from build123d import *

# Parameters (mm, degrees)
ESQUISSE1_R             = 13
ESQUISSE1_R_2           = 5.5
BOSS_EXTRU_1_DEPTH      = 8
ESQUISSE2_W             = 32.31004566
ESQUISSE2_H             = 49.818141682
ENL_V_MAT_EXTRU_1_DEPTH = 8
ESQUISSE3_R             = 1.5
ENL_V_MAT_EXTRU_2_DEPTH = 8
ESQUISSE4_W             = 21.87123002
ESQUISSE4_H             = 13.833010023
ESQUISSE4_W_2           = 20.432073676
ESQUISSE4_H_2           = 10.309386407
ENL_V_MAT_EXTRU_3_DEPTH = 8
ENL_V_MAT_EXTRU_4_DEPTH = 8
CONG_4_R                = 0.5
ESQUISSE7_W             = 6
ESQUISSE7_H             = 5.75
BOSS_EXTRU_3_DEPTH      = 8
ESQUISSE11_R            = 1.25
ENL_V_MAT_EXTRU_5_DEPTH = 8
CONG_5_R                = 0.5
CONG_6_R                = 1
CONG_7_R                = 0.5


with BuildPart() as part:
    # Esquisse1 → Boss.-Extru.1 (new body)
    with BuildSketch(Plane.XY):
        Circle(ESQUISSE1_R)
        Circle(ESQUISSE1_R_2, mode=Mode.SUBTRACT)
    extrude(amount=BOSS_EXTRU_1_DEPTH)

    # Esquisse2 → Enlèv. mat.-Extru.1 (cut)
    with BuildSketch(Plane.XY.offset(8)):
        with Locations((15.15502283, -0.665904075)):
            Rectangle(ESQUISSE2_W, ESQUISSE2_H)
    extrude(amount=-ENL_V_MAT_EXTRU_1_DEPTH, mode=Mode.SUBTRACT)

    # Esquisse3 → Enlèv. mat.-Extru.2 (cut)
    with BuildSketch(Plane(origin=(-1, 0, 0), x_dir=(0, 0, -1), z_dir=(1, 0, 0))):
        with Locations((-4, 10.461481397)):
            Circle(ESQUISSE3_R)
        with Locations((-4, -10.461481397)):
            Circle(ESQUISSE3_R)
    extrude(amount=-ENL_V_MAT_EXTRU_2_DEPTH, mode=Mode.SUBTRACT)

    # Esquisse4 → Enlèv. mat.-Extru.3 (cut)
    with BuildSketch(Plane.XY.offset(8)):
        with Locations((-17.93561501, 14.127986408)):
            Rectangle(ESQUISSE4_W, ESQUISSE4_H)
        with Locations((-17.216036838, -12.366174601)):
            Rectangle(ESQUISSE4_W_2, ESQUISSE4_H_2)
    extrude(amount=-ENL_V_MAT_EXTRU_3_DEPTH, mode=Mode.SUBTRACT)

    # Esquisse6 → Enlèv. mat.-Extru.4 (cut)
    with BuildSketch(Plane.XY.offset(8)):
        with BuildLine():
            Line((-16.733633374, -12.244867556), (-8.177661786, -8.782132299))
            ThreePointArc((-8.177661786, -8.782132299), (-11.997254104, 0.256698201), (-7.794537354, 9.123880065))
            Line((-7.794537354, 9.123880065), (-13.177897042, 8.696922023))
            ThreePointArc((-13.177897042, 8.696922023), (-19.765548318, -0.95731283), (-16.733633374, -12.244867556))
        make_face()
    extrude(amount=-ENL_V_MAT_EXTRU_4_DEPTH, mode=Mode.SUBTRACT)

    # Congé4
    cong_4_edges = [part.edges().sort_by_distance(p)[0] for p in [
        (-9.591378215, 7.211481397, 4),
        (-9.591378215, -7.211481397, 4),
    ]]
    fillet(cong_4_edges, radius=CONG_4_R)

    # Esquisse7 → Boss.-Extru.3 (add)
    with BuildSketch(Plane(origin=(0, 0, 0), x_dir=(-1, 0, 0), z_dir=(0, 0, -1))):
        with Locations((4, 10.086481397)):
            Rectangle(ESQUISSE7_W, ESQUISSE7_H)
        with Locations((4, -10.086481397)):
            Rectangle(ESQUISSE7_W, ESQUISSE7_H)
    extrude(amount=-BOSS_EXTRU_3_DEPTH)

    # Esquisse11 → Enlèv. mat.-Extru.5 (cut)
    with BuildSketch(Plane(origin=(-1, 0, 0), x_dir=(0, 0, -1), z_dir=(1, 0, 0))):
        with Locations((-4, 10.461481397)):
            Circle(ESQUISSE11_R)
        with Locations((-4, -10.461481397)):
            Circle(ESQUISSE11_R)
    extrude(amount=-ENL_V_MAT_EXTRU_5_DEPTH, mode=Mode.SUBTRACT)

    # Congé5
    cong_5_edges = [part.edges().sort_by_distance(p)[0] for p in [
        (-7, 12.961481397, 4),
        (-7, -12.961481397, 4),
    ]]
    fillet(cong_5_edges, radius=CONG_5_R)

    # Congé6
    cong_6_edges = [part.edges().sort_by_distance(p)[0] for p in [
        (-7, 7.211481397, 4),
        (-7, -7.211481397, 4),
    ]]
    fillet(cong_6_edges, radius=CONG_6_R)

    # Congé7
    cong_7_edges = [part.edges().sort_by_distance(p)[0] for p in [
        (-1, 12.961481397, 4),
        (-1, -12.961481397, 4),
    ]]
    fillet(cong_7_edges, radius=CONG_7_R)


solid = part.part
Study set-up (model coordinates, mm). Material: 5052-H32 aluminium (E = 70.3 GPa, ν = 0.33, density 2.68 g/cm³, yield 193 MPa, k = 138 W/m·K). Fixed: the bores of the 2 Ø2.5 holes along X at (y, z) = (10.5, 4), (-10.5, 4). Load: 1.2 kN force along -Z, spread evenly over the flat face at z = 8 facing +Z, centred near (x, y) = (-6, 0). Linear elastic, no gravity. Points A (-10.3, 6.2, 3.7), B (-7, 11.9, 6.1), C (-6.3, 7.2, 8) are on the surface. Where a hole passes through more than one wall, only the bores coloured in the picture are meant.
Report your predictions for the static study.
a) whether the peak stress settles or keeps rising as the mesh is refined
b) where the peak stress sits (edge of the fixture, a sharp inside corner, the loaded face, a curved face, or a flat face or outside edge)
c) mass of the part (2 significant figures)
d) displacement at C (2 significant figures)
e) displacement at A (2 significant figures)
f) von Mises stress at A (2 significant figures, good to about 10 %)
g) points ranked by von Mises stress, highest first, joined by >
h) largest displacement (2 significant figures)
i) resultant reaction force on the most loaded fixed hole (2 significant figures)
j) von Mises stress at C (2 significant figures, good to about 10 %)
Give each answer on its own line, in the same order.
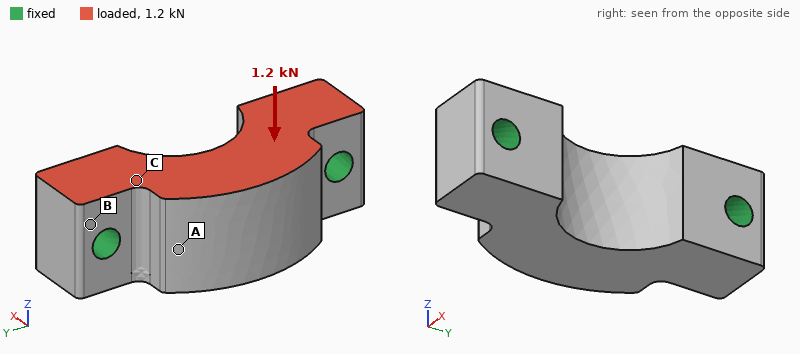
keeps rising
edge of the fixture
3.7 g
4.6 µm
7.7 µm
18 MPa
C > A > B
12 µm
600 N
33 MPa
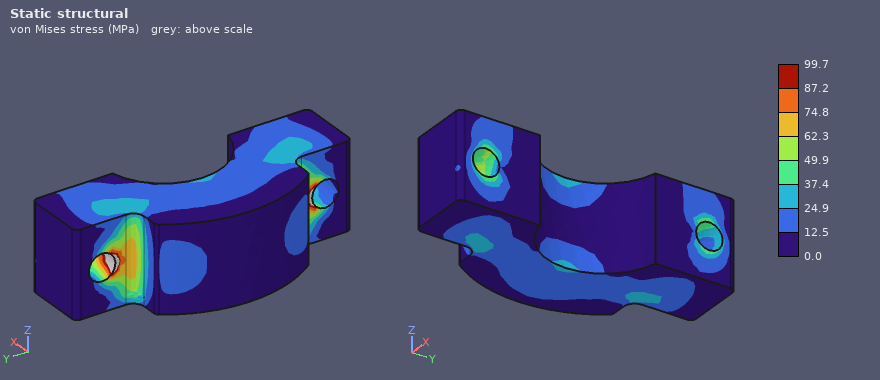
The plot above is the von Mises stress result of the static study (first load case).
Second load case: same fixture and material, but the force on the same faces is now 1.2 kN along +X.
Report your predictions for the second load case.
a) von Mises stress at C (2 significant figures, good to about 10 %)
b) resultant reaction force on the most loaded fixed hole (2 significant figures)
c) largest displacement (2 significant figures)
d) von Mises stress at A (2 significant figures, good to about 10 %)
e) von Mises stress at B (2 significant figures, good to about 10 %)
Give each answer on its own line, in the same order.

46 MPa
640 N
13 µm
14 MPa
17 MPa
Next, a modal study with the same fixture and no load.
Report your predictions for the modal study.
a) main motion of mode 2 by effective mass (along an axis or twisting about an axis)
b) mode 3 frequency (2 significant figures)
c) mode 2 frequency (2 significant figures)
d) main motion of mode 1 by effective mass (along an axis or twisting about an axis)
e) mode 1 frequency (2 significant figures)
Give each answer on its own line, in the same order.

along X
73 kHz
55 kHz
along Z
32 kHz
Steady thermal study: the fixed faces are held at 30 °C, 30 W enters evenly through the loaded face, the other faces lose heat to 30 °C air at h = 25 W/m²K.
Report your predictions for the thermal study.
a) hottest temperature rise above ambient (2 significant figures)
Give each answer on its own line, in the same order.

15 K
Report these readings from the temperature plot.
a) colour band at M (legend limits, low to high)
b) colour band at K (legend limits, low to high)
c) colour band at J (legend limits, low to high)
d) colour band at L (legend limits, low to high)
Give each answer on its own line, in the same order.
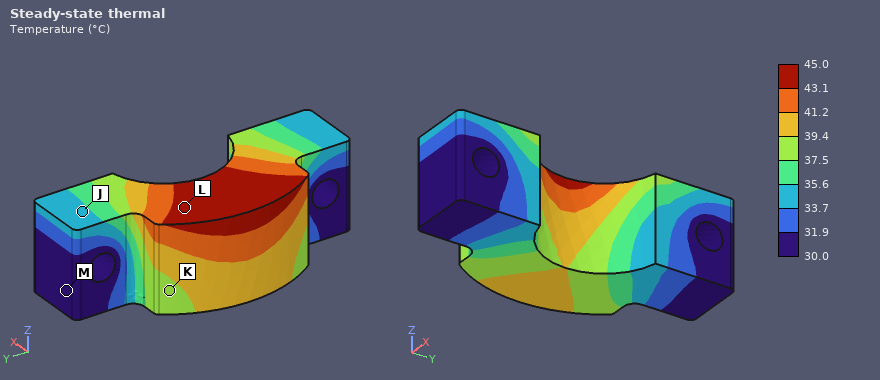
30.0 to 31.9 °C
37.5 to 39.4 °C
33.7 to 35.6 °C
43.1 to 45.0 °C
